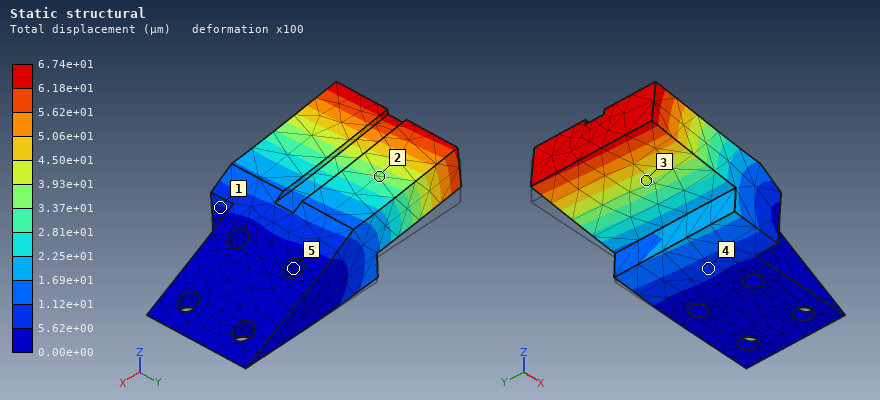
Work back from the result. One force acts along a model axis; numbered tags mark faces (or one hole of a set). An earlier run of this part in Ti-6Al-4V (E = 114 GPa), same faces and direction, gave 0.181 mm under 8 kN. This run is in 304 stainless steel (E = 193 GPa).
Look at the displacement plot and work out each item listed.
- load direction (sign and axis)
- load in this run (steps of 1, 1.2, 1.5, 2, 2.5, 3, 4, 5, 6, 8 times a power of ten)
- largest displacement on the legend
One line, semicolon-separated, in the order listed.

+Z; 5 kN; 6.74e+01 µm
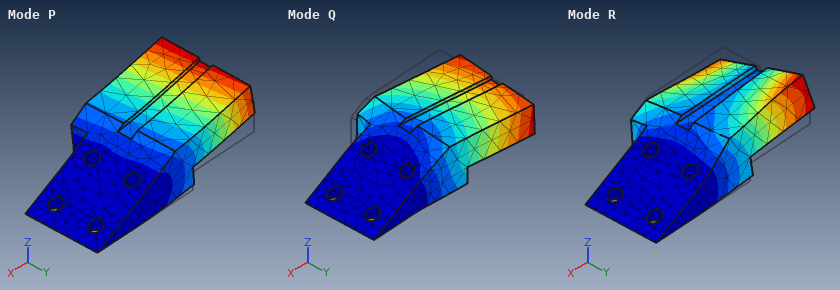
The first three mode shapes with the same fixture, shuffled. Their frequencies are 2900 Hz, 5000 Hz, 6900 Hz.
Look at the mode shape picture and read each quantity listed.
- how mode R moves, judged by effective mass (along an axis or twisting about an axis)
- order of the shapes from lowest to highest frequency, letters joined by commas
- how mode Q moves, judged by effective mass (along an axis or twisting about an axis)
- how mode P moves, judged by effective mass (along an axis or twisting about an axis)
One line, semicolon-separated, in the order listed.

twisting about X; P, Q, R; along Y; along Z
